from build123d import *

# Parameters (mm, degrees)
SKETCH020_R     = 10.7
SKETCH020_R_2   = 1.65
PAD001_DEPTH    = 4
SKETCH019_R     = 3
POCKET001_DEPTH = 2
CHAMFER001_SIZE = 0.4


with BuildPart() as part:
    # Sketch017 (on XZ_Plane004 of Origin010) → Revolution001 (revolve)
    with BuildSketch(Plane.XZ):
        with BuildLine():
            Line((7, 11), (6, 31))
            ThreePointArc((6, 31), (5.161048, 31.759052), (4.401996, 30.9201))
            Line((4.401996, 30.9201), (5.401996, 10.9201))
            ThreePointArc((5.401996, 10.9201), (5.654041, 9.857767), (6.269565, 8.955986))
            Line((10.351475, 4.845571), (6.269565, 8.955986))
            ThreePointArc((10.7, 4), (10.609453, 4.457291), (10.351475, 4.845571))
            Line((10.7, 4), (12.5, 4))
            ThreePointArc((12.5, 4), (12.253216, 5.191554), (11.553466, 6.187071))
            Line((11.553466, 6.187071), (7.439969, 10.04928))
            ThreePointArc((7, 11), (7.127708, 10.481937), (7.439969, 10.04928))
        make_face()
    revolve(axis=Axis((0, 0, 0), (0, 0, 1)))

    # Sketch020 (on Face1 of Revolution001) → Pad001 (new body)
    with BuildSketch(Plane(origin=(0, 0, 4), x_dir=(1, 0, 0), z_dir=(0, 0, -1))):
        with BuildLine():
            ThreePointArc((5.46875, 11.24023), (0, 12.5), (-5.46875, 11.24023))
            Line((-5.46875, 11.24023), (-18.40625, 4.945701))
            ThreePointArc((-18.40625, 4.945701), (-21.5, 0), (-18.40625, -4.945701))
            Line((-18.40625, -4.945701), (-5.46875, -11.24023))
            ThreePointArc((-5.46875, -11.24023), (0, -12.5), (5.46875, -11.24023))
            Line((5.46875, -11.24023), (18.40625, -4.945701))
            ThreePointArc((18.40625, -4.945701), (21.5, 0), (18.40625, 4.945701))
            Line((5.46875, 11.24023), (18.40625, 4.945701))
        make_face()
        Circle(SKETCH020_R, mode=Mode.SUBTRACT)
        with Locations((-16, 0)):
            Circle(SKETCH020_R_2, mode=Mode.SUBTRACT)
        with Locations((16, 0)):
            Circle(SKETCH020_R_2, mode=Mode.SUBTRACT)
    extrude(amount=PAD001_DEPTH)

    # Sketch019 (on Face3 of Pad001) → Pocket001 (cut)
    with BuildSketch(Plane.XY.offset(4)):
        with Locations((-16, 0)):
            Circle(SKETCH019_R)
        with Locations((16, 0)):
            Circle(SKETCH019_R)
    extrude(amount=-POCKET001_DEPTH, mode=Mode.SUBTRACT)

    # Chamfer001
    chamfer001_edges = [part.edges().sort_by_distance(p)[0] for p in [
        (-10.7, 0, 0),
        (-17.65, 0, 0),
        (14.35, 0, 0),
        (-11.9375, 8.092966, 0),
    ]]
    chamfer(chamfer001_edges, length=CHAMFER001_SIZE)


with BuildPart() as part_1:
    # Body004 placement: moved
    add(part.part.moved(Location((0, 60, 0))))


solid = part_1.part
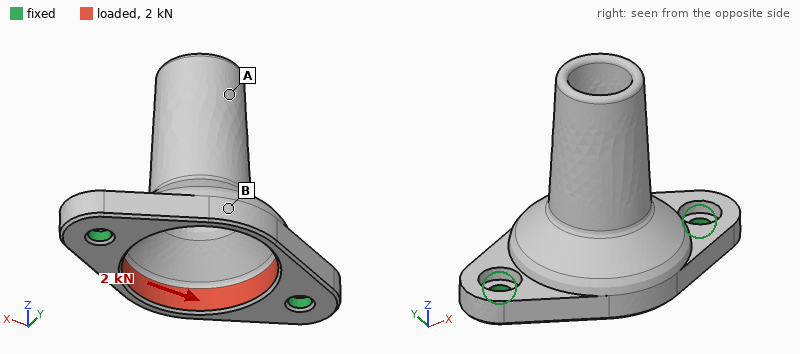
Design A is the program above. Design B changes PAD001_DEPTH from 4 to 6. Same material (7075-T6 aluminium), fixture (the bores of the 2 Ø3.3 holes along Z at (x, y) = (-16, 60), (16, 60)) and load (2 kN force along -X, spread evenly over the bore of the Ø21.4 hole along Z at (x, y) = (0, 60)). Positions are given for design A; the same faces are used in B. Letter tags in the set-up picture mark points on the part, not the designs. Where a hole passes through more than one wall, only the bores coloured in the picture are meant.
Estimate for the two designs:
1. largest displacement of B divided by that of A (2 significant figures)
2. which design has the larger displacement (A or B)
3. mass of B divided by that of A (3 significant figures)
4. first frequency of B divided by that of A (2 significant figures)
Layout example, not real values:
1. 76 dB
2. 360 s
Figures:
1. 0.66
2. A
3. 1.21
4. 1.6
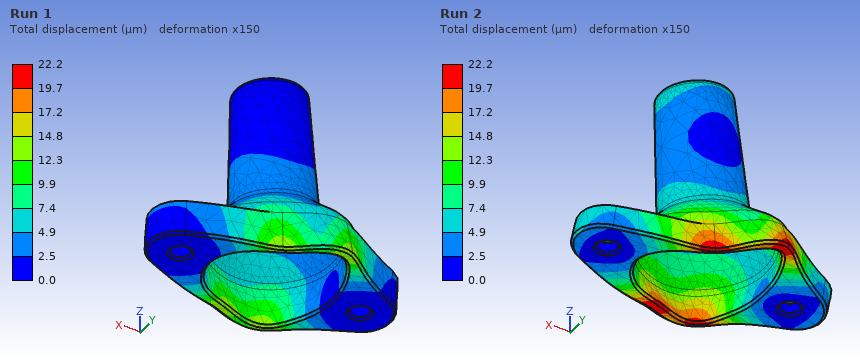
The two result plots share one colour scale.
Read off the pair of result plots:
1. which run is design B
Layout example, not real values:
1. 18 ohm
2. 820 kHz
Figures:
1. Run 1
